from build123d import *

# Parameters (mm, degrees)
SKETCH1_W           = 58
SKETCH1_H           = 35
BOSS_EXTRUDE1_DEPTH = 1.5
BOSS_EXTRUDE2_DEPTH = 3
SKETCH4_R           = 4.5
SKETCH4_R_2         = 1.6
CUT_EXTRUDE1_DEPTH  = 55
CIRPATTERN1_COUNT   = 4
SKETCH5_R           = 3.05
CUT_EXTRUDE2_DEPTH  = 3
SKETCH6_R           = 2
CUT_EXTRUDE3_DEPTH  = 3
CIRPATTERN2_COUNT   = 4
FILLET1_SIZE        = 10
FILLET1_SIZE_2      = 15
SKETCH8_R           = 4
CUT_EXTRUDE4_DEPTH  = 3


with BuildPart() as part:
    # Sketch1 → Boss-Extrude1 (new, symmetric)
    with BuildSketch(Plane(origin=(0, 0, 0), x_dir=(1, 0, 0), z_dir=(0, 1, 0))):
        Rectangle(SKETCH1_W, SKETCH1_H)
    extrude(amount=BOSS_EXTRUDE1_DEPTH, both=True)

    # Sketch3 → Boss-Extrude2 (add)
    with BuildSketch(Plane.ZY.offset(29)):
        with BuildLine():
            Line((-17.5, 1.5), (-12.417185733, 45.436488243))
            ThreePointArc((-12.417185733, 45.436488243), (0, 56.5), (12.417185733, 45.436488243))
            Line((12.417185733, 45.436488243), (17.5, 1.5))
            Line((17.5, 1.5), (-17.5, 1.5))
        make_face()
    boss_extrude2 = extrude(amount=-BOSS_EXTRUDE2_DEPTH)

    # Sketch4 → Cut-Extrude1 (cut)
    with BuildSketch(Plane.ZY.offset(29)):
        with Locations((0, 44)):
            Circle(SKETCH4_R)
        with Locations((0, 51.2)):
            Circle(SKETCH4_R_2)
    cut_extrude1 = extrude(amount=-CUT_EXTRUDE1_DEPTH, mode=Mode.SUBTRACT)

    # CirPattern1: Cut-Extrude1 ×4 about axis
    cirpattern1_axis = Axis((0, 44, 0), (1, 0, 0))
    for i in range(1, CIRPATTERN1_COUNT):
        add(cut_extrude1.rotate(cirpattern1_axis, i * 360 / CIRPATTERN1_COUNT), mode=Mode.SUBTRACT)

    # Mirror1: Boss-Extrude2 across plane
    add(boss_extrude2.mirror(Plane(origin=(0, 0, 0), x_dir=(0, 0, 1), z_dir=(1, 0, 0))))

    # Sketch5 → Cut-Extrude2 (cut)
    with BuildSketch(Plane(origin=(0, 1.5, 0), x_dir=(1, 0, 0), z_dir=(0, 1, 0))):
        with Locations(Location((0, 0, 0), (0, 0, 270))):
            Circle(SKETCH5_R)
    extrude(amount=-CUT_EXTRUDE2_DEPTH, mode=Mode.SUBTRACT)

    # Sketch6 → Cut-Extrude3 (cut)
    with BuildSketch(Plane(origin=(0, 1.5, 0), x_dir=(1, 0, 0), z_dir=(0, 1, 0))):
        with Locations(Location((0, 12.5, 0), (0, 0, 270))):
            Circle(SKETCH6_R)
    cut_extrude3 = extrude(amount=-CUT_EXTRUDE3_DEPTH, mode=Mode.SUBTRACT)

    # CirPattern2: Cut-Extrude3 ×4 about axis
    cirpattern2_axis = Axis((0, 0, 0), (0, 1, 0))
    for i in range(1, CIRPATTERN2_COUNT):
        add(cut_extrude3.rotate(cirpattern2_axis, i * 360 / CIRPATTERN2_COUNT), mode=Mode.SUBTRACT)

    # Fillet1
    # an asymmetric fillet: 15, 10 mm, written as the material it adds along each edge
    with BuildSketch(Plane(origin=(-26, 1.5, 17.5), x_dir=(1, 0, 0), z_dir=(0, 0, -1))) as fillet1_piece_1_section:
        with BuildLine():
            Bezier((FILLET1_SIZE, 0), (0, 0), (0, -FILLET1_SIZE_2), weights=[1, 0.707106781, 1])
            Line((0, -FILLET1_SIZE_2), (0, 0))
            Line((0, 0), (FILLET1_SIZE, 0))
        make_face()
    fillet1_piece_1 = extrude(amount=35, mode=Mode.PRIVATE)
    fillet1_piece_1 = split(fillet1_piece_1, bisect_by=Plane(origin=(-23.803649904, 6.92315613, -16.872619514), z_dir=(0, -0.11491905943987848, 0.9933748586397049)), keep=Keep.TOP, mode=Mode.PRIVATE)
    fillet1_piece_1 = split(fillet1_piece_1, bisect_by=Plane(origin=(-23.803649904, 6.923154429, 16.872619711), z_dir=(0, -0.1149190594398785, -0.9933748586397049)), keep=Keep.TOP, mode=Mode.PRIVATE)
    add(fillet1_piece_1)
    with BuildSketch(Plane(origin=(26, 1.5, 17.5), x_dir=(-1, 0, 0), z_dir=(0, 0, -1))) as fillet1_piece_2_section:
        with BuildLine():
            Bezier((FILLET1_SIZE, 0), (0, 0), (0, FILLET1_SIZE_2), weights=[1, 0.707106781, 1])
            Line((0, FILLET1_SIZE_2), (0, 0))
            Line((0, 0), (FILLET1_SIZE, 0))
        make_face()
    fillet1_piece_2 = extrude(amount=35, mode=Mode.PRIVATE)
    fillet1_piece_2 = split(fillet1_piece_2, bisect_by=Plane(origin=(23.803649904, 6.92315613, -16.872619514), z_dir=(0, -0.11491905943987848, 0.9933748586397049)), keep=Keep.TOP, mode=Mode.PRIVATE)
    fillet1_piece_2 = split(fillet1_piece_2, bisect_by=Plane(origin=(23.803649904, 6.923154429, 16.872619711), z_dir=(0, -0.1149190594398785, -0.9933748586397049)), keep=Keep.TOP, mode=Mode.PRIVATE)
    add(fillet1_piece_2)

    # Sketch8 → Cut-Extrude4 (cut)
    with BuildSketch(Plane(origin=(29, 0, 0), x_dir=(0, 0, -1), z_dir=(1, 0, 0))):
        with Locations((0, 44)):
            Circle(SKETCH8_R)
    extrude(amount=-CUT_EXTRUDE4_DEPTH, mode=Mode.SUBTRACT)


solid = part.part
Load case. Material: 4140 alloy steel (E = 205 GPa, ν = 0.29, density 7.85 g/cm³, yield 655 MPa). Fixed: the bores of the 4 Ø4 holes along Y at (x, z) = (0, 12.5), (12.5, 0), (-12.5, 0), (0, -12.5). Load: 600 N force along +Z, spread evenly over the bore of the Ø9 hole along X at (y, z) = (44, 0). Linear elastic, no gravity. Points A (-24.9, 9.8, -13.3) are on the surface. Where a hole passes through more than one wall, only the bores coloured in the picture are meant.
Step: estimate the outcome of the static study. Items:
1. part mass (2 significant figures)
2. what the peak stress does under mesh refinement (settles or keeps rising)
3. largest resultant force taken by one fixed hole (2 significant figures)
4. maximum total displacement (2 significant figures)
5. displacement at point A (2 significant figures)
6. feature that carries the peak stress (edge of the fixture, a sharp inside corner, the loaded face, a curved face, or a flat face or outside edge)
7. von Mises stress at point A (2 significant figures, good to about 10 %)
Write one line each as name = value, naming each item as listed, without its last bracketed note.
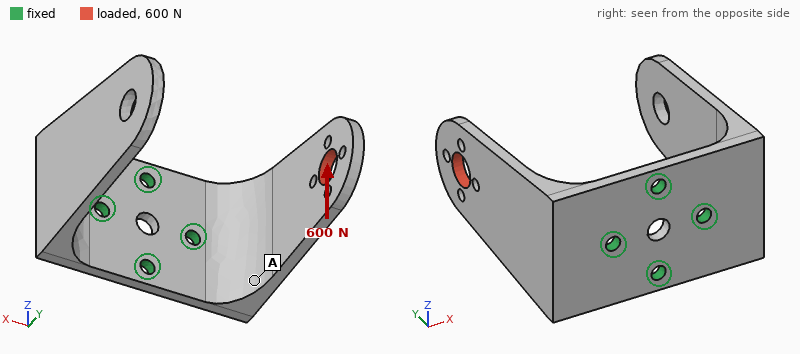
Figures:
part mass = 130 g
what the peak stress does under mesh refinement = keeps rising
largest resultant force taken by one fixed hole = 560 N
maximum total displacement = 0.36 mm
displacement at point A = 0.098 mm
feature that carries the peak stress = edge of the fixture
von Mises stress at point A = 67 MPa
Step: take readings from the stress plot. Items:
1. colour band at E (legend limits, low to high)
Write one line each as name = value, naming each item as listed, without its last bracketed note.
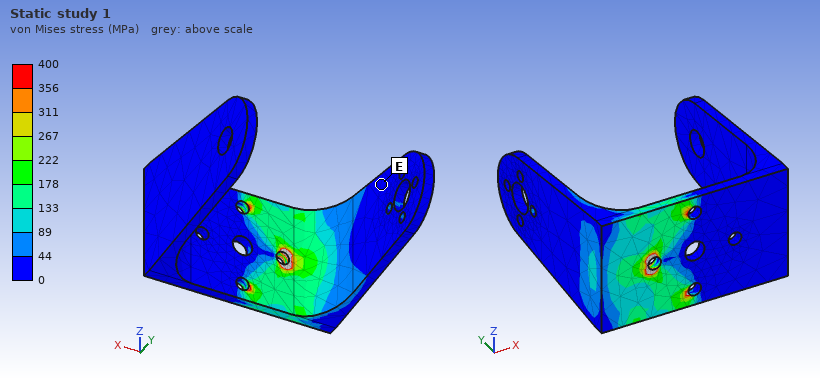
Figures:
colour band at E = 0 to 44 MPa
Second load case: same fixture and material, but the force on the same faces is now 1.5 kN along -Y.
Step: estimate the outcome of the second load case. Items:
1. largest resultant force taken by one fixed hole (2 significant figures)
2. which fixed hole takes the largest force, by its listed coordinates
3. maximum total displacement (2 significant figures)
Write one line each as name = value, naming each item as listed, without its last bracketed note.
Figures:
largest resultant force taken by one fixed hole = 2.2 kN
which fixed hole takes the largest force, by its listed coordinates = (-12.5, 0)
maximum total displacement = 0.49 mm
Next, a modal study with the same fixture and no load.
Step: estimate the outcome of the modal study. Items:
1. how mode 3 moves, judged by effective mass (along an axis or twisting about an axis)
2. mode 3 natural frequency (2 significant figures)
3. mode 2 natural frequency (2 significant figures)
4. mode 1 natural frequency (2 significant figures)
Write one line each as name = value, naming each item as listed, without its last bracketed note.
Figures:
how mode 3 moves, judged by effective mass = along Z
mode 3 natural frequency = 1800 Hz
mode 2 natural frequency = 990 Hz
mode 1 natural frequency = 960 Hz
